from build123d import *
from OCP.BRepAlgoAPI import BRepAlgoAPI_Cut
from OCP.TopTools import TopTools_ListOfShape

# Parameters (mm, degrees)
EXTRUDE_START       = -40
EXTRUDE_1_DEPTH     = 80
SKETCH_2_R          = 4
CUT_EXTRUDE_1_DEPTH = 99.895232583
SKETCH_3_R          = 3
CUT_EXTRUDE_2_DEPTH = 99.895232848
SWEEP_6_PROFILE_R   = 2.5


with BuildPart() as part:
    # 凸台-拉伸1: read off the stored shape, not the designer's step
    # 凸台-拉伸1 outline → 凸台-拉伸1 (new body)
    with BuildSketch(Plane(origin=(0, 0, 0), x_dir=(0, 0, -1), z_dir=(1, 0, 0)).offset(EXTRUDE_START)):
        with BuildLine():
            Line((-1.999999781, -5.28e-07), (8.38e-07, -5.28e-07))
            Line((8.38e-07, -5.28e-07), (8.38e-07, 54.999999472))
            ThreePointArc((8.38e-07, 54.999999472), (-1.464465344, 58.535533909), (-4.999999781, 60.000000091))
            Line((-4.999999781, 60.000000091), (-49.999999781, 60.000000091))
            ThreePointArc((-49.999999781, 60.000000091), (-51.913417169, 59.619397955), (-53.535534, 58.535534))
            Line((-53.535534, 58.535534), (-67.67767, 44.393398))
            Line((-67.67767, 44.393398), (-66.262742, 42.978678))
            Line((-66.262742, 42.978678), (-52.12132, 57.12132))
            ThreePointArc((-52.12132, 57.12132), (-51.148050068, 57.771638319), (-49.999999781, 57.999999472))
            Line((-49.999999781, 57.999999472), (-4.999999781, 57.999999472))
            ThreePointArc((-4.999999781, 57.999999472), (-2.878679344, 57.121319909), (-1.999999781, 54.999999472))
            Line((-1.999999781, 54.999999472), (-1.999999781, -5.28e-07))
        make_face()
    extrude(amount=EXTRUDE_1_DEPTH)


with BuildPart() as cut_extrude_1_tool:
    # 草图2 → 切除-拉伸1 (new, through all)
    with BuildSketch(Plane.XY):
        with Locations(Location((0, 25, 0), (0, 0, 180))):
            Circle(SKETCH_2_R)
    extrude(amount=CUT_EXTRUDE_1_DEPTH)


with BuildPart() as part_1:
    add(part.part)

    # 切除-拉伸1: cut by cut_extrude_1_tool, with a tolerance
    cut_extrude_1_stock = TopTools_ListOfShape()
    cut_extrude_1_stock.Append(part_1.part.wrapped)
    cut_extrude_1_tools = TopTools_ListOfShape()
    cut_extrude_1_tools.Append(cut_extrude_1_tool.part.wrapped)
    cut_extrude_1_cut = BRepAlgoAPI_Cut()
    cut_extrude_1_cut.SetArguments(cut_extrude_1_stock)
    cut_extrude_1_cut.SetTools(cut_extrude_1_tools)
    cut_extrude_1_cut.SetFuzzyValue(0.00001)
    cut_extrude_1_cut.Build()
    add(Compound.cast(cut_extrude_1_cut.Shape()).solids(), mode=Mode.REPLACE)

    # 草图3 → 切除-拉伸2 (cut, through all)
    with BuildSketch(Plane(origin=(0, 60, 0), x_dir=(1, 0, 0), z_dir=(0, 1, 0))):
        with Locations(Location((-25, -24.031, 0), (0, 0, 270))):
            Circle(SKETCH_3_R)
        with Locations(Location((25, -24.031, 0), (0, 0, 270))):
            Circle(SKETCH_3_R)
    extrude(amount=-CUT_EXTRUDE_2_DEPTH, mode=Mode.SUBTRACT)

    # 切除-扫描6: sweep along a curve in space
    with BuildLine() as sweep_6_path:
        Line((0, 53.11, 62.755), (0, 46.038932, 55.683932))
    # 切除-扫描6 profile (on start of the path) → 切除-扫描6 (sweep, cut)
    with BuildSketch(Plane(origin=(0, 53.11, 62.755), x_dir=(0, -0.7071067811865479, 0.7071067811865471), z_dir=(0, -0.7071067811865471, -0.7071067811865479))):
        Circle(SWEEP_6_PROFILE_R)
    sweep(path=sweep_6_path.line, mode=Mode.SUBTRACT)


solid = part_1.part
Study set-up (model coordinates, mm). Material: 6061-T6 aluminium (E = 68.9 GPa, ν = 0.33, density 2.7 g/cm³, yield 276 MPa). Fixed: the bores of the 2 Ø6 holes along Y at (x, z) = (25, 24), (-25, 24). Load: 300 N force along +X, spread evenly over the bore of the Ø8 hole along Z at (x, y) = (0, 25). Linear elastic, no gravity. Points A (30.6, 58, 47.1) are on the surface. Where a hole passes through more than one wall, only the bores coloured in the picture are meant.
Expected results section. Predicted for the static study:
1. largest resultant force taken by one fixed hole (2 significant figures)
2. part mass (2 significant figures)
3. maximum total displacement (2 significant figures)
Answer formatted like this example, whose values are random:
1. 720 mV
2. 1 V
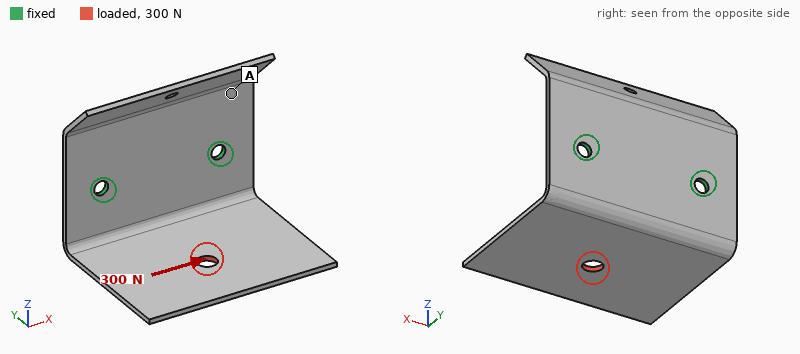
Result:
1. 270 N
2. 55 g
3. 0.74 mm
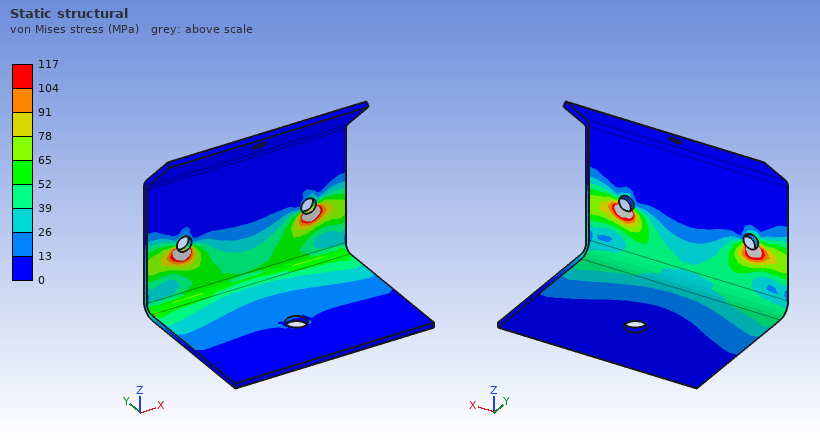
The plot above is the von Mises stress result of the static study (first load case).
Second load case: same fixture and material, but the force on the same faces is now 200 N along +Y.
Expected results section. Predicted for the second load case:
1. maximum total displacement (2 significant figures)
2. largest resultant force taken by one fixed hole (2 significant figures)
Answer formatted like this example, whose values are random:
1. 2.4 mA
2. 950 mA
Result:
1. 0.84 mm
2. 100 N
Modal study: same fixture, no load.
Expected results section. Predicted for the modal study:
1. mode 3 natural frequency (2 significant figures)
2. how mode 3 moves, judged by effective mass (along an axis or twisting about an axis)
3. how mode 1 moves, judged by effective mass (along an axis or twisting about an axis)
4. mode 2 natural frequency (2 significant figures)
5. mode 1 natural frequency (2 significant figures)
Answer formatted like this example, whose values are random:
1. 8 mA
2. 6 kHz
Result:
1. 740 Hz
2. along Y
3. along Z
4. 670 Hz
5. 300 Hz
